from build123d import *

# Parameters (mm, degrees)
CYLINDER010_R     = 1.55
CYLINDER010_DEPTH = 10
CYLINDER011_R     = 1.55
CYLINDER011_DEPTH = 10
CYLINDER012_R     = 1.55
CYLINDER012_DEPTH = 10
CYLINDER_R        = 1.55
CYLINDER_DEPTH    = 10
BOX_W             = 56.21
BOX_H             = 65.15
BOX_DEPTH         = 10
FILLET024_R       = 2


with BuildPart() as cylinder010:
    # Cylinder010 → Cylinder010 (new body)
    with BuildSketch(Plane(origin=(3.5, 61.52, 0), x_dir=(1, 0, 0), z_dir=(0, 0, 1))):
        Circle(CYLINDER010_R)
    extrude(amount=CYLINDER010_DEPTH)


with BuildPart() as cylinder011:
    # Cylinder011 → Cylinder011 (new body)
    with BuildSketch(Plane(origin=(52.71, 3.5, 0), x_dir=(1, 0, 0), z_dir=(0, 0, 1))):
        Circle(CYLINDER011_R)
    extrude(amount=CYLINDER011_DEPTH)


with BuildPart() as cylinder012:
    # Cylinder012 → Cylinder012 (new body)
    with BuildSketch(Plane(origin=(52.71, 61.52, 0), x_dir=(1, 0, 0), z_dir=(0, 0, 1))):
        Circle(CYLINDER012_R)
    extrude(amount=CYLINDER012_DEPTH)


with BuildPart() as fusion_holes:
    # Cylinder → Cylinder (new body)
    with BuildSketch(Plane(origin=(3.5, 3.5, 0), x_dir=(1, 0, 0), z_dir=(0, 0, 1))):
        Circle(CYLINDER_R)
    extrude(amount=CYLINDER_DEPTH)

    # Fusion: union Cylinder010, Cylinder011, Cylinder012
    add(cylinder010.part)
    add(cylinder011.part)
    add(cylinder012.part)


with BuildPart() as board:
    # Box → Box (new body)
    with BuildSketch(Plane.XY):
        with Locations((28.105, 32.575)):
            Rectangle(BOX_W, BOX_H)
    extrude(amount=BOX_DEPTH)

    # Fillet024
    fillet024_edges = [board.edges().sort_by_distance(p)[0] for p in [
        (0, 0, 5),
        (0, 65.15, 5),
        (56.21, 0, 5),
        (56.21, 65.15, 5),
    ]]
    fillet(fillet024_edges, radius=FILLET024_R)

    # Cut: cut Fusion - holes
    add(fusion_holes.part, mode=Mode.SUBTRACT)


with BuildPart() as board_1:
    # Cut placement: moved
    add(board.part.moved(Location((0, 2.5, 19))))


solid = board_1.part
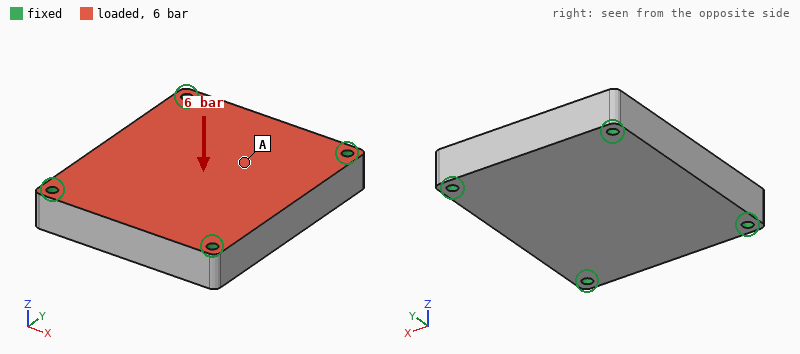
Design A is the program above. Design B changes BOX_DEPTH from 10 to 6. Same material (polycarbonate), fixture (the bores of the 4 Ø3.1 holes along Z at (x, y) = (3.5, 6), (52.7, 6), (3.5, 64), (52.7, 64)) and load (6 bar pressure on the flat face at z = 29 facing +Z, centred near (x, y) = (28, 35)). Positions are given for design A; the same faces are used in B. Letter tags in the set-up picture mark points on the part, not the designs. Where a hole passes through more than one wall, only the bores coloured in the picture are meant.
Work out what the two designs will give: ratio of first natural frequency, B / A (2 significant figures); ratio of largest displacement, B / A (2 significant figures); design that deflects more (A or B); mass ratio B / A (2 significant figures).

0.68
3.8
B
0.60
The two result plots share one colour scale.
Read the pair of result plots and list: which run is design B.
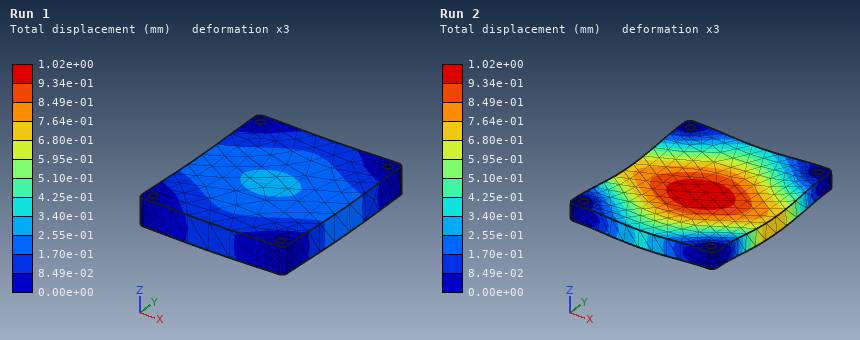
Run 2
